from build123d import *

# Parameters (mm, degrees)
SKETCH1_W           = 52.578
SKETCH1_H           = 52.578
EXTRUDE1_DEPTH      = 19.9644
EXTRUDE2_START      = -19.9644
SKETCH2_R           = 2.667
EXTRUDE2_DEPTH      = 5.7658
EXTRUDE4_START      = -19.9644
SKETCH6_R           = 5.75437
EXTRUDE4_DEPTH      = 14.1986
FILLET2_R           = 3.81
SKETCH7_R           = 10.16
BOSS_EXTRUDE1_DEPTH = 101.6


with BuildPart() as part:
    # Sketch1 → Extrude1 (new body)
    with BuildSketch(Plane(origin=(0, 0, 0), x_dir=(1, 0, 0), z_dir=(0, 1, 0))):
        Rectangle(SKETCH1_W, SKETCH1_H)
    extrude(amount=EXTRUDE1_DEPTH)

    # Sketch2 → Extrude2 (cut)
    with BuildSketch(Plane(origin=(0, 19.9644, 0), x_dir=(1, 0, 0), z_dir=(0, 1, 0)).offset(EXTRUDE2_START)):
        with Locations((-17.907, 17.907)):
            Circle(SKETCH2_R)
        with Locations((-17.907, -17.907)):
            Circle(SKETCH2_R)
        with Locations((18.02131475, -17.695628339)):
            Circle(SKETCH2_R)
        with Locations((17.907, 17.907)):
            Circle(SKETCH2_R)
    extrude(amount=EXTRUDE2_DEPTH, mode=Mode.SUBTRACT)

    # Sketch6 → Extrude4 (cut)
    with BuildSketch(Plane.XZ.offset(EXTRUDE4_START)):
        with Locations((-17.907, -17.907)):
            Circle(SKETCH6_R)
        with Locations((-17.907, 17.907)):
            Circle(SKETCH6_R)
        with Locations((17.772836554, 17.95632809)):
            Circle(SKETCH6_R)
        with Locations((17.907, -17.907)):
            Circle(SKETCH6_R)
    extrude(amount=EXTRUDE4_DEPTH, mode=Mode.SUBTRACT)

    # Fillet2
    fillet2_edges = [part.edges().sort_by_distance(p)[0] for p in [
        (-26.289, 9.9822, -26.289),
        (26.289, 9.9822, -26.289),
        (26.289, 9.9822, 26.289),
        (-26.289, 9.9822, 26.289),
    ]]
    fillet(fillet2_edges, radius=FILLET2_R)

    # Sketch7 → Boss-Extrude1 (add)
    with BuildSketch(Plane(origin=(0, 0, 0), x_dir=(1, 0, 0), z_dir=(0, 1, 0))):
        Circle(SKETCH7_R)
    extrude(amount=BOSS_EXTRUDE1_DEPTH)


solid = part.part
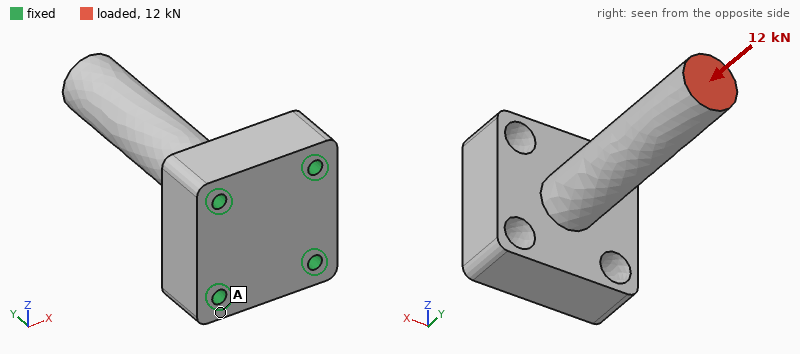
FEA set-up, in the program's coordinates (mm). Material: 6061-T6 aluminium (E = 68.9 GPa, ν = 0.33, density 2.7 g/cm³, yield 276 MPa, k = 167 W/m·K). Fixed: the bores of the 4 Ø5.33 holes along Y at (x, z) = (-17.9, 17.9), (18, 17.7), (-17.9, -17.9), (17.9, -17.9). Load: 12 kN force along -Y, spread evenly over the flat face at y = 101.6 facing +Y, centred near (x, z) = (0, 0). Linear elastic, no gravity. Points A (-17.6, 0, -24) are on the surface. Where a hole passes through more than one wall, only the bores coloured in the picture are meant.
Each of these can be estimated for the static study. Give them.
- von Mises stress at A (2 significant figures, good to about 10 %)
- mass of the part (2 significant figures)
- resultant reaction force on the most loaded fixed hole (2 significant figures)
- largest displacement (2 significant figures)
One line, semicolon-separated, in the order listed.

18 MPa; 200 g; 3.3 kN; 58 µm
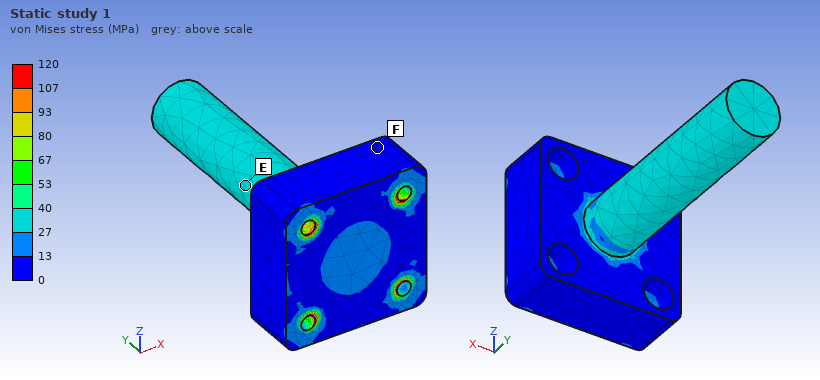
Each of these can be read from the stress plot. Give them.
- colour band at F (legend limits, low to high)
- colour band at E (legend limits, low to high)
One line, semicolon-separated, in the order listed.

0 to 13 MPa; 27 to 40 MPa
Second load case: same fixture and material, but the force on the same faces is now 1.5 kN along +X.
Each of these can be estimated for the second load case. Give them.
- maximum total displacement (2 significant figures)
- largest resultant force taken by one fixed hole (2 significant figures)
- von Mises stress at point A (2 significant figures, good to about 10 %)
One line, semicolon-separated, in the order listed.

0.61 mm; 2.2 kN; 9.6 MPa
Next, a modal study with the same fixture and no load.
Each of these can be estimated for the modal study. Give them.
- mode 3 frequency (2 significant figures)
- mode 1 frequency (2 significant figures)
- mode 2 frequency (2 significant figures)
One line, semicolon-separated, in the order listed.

9100 Hz; 1800 Hz; 1800 Hz
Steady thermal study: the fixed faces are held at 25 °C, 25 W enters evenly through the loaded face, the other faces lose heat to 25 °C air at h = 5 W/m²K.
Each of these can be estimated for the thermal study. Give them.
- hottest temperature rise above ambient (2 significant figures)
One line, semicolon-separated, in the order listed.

42 K
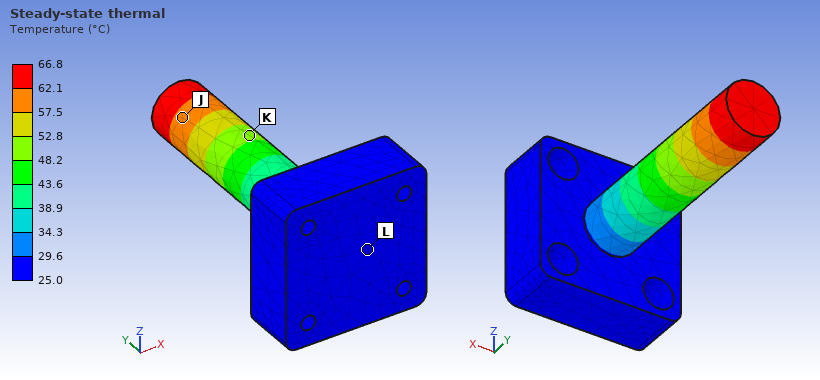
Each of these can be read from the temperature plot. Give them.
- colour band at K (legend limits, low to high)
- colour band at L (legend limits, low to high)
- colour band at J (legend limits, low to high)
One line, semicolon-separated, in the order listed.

48.2 to 52.8 °C; 25.0 to 29.6 °C; 57.5 to 62.1 °C
